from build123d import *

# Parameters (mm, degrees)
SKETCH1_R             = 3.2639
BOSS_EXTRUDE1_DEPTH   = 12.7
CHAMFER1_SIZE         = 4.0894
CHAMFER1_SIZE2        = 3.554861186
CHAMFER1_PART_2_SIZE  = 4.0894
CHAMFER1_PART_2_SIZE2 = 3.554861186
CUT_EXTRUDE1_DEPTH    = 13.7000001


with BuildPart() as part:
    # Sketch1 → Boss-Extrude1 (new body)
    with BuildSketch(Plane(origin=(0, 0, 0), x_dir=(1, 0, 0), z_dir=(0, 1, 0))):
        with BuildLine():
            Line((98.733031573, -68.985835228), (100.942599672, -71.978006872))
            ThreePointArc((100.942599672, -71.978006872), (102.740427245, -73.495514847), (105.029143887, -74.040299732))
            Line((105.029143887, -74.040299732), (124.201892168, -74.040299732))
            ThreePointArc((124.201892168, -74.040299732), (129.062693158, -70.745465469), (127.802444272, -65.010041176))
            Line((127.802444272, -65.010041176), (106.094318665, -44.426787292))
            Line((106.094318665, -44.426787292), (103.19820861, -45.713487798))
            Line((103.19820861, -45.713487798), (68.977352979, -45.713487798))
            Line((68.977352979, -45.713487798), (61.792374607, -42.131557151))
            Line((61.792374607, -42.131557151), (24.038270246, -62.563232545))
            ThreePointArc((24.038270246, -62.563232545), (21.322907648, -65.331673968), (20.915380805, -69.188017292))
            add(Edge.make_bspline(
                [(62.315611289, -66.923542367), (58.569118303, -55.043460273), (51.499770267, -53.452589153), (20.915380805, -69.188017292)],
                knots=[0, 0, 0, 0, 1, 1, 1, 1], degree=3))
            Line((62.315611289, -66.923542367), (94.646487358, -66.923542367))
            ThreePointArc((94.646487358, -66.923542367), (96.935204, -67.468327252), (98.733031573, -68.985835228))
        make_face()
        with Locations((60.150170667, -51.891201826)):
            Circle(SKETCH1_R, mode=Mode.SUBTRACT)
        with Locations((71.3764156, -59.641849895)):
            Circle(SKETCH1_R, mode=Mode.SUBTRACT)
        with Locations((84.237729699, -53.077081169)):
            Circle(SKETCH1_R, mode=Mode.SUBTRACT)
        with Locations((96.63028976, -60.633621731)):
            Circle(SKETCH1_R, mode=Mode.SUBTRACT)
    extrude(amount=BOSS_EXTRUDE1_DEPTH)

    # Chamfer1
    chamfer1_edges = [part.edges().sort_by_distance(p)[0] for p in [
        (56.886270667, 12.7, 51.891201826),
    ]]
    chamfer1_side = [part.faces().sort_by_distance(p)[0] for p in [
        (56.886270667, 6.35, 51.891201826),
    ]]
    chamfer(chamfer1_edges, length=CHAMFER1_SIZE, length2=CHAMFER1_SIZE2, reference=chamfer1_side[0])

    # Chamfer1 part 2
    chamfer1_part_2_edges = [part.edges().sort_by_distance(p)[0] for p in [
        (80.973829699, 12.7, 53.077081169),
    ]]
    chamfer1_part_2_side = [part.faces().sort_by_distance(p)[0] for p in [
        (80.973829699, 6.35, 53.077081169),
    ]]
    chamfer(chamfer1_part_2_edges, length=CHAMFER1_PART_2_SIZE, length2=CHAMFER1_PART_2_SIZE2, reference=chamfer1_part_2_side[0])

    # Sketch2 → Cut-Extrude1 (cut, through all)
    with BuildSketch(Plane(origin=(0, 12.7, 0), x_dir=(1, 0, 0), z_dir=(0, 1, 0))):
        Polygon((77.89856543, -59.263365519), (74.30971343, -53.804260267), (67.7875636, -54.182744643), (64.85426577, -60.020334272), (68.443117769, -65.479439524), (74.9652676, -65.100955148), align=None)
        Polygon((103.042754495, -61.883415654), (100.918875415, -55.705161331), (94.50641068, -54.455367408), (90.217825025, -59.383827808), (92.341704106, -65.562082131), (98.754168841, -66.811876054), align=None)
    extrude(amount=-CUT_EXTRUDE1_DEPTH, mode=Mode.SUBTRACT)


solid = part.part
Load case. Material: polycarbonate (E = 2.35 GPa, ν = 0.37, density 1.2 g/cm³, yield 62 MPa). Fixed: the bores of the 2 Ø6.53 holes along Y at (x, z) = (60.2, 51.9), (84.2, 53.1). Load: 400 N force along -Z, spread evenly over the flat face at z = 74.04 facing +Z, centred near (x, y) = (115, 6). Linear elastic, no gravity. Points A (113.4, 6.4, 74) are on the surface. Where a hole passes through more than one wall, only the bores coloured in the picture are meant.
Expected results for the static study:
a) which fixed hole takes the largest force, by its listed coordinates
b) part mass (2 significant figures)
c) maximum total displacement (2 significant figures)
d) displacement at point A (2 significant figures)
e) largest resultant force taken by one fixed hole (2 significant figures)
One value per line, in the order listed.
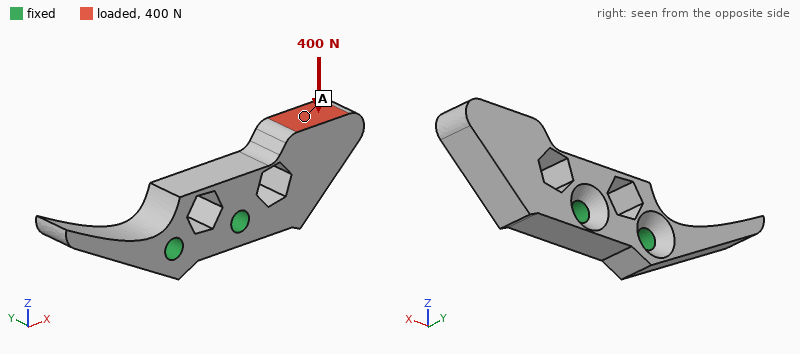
(84.2, 53.1)
22 g
0.93 mm
0.69 mm
570 N
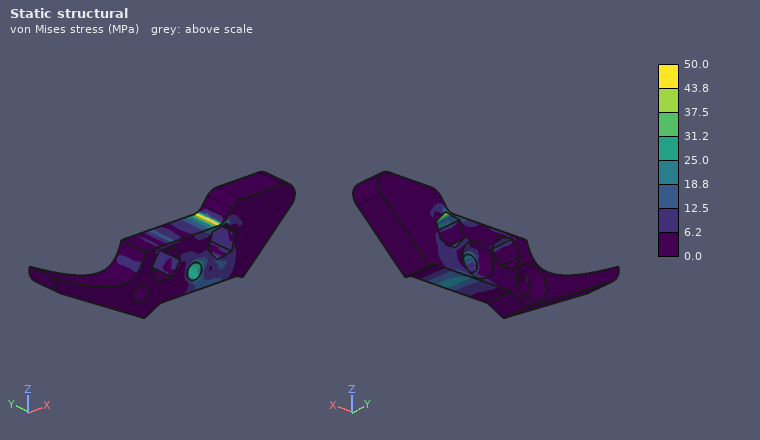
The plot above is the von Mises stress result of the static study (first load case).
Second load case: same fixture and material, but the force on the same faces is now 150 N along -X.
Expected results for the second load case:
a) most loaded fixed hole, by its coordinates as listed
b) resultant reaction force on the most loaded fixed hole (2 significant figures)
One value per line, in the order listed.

(84.2, 53.1)
140 N
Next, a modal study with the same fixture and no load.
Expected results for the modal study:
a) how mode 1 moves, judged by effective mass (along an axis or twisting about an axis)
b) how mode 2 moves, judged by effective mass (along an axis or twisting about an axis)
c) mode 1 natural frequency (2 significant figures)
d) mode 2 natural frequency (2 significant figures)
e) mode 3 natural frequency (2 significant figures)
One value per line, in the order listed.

along Y
along Z
980 Hz
1300 Hz
1500 Hz
